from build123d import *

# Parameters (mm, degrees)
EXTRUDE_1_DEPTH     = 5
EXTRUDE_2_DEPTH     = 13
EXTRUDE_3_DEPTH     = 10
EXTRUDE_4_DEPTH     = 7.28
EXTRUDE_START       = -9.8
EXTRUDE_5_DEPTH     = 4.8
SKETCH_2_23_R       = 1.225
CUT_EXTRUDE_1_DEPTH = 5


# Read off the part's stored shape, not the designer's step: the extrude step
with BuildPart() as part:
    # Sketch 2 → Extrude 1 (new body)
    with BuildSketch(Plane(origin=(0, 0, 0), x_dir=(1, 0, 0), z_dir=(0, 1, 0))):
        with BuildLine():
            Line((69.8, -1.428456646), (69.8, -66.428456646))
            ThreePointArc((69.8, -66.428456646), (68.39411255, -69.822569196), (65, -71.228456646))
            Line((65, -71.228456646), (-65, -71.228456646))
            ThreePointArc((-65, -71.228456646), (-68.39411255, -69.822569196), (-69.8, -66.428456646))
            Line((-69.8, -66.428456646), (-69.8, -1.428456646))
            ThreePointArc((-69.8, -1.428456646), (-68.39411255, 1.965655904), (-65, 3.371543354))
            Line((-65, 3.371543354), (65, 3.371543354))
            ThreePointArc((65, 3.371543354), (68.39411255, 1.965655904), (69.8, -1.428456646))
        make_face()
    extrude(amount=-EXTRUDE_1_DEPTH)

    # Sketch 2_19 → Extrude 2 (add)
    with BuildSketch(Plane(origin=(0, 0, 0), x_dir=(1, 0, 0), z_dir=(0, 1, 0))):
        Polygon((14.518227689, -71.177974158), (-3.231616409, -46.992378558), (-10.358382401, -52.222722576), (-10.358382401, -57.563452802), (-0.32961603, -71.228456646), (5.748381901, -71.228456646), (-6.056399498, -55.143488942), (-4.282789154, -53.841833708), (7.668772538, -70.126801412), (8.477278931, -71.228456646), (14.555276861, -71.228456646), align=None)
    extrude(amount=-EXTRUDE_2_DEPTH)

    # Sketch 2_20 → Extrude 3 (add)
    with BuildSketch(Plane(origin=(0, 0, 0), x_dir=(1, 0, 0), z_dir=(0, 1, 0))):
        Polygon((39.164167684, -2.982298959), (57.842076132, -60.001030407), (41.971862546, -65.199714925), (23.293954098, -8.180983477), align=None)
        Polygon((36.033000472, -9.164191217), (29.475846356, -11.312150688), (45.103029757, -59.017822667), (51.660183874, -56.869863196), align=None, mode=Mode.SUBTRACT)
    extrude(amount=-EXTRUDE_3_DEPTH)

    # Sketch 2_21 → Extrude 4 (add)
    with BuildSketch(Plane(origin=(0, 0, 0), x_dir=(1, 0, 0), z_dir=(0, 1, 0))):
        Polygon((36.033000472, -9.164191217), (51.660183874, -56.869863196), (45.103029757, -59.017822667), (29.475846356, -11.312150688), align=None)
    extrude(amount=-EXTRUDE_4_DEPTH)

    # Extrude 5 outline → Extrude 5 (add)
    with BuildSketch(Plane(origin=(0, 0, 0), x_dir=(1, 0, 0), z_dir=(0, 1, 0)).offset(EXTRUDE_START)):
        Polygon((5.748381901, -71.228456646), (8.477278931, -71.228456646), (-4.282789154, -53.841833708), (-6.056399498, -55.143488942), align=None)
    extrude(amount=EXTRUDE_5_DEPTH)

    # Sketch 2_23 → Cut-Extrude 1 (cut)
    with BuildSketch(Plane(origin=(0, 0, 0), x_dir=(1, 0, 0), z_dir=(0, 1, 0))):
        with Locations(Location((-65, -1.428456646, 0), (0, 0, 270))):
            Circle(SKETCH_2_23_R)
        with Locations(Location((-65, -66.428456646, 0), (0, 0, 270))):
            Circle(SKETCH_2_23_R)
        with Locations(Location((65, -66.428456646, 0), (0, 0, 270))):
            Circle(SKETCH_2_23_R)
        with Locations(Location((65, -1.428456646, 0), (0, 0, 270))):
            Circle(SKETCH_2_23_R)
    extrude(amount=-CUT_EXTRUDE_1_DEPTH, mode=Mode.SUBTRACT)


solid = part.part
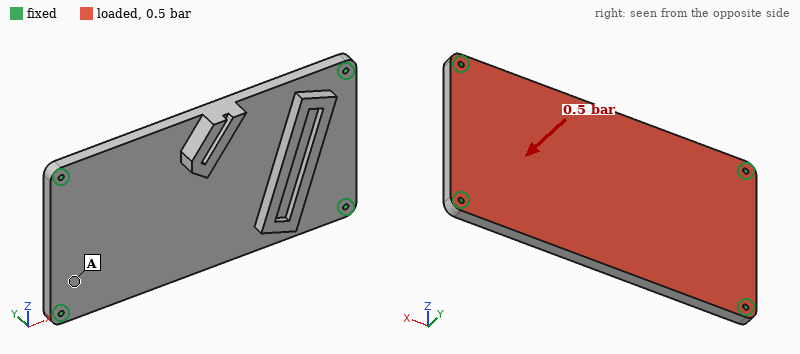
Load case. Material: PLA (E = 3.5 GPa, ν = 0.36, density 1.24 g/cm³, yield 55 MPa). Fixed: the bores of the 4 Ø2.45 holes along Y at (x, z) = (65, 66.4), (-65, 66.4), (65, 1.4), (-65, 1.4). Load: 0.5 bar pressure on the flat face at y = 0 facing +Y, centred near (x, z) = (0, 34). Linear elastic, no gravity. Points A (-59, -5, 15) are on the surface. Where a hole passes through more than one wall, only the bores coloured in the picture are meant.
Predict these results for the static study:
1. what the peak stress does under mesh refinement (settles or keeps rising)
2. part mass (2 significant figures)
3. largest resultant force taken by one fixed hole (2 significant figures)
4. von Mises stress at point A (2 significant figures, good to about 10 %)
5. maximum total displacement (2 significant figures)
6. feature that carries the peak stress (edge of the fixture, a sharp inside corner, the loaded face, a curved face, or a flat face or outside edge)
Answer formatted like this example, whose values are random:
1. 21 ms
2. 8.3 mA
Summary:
1. keeps rising
2. 72 g
3. 130 N
4. 6.4 MPa
5. 1.7 mm
6. edge of the fixture
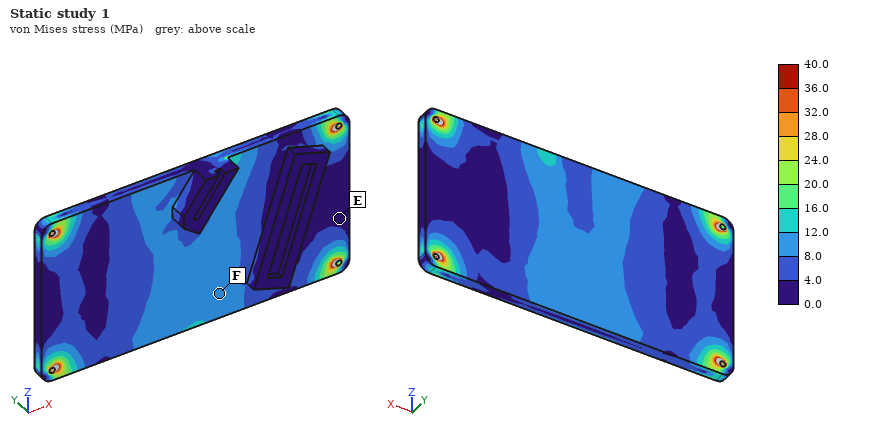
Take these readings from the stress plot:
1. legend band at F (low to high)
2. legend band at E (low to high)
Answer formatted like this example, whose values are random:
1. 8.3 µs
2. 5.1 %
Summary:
1. 8.0 to 12.0 MPa
2. 0.0 to 4.0 MPa
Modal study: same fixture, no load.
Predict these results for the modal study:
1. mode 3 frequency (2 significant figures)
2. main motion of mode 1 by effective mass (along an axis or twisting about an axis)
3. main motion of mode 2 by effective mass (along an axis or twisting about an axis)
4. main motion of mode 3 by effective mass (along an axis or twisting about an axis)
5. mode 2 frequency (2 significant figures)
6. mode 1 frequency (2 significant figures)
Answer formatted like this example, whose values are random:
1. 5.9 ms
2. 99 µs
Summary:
1. 1100 Hz
2. along Y
3. twisting about X
4. twisting about Z
5. 750 Hz
6. 380 Hz
